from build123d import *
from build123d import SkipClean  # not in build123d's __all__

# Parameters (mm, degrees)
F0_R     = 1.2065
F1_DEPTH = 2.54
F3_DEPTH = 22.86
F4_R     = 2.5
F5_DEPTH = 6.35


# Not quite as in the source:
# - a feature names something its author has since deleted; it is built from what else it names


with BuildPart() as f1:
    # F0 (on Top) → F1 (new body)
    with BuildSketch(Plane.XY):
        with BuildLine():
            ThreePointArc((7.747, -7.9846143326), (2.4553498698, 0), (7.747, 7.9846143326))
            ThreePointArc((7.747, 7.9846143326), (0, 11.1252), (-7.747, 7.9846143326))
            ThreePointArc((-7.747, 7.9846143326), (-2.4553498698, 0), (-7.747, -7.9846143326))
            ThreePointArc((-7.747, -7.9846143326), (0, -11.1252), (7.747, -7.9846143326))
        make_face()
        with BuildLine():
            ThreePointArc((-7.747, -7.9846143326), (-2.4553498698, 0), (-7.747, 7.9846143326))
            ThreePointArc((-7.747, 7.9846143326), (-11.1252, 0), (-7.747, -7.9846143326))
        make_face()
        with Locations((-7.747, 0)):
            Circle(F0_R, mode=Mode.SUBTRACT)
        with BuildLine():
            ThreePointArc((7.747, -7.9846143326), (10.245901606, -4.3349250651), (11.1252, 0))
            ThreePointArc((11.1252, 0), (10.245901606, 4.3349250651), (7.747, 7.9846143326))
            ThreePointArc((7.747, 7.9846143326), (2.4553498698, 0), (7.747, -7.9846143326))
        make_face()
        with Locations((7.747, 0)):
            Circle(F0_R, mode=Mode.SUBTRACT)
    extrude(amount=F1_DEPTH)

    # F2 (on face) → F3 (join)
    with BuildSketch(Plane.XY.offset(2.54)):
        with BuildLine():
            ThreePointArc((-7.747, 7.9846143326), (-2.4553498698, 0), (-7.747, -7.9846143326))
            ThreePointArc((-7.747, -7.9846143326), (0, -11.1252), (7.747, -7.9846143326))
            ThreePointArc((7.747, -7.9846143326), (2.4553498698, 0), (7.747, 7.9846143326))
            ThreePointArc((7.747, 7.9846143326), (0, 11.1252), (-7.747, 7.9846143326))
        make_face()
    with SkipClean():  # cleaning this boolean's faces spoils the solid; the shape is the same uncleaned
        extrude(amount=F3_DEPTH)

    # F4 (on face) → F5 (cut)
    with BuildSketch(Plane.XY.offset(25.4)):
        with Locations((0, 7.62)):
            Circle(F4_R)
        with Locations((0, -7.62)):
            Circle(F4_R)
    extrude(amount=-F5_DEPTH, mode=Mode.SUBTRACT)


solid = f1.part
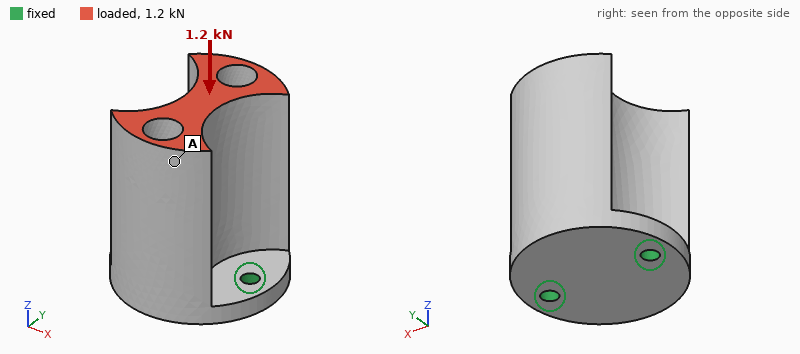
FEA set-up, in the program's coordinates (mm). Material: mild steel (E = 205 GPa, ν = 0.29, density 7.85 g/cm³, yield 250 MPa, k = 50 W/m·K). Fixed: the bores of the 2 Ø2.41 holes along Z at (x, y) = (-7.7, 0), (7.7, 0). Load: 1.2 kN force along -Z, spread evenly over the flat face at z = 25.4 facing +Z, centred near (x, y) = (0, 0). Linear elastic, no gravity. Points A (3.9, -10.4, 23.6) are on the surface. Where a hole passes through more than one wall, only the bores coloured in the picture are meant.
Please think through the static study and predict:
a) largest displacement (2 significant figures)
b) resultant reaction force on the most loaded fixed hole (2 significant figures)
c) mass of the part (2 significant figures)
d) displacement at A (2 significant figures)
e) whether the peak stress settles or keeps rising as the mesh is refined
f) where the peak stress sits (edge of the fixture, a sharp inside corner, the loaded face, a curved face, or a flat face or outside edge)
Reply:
5.1 µm
620 N
40 g
5.0 µm
keeps rising
edge of the fixture
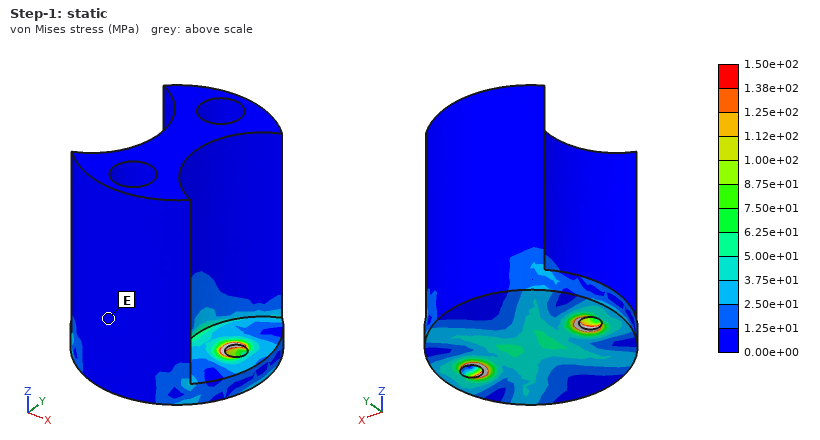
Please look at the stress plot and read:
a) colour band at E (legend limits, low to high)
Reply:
0.00e+00 to 1.25e+01 MPa
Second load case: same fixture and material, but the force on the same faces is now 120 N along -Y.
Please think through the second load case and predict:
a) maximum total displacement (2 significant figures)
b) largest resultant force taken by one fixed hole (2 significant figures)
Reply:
24 µm
60 N
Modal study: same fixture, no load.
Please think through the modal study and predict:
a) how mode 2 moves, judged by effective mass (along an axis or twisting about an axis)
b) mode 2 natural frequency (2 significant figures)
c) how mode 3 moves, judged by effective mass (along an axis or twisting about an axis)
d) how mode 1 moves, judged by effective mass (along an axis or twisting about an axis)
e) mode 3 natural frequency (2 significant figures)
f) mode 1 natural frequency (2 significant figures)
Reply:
along X
5900 Hz
along Z
along Y
13 kHz
3200 Hz
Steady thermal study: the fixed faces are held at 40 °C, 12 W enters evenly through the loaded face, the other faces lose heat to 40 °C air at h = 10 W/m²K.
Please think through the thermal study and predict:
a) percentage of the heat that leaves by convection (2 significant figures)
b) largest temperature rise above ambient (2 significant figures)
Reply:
6.6 %
50 K
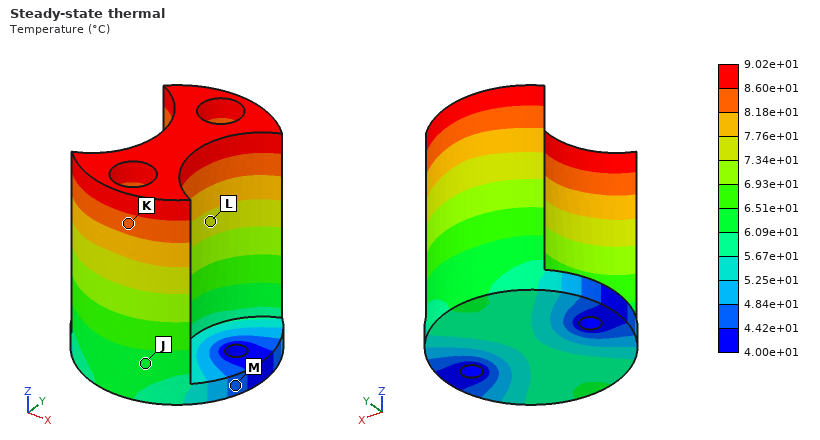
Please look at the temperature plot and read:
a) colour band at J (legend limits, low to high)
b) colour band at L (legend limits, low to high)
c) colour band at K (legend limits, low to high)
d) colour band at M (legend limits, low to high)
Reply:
6.09e+01 to 6.51e+01 °C
7.34e+01 to 7.76e+01 °C
8.18e+01 to 8.60e+01 °C
4.42e+01 to 4.84e+01 °C
